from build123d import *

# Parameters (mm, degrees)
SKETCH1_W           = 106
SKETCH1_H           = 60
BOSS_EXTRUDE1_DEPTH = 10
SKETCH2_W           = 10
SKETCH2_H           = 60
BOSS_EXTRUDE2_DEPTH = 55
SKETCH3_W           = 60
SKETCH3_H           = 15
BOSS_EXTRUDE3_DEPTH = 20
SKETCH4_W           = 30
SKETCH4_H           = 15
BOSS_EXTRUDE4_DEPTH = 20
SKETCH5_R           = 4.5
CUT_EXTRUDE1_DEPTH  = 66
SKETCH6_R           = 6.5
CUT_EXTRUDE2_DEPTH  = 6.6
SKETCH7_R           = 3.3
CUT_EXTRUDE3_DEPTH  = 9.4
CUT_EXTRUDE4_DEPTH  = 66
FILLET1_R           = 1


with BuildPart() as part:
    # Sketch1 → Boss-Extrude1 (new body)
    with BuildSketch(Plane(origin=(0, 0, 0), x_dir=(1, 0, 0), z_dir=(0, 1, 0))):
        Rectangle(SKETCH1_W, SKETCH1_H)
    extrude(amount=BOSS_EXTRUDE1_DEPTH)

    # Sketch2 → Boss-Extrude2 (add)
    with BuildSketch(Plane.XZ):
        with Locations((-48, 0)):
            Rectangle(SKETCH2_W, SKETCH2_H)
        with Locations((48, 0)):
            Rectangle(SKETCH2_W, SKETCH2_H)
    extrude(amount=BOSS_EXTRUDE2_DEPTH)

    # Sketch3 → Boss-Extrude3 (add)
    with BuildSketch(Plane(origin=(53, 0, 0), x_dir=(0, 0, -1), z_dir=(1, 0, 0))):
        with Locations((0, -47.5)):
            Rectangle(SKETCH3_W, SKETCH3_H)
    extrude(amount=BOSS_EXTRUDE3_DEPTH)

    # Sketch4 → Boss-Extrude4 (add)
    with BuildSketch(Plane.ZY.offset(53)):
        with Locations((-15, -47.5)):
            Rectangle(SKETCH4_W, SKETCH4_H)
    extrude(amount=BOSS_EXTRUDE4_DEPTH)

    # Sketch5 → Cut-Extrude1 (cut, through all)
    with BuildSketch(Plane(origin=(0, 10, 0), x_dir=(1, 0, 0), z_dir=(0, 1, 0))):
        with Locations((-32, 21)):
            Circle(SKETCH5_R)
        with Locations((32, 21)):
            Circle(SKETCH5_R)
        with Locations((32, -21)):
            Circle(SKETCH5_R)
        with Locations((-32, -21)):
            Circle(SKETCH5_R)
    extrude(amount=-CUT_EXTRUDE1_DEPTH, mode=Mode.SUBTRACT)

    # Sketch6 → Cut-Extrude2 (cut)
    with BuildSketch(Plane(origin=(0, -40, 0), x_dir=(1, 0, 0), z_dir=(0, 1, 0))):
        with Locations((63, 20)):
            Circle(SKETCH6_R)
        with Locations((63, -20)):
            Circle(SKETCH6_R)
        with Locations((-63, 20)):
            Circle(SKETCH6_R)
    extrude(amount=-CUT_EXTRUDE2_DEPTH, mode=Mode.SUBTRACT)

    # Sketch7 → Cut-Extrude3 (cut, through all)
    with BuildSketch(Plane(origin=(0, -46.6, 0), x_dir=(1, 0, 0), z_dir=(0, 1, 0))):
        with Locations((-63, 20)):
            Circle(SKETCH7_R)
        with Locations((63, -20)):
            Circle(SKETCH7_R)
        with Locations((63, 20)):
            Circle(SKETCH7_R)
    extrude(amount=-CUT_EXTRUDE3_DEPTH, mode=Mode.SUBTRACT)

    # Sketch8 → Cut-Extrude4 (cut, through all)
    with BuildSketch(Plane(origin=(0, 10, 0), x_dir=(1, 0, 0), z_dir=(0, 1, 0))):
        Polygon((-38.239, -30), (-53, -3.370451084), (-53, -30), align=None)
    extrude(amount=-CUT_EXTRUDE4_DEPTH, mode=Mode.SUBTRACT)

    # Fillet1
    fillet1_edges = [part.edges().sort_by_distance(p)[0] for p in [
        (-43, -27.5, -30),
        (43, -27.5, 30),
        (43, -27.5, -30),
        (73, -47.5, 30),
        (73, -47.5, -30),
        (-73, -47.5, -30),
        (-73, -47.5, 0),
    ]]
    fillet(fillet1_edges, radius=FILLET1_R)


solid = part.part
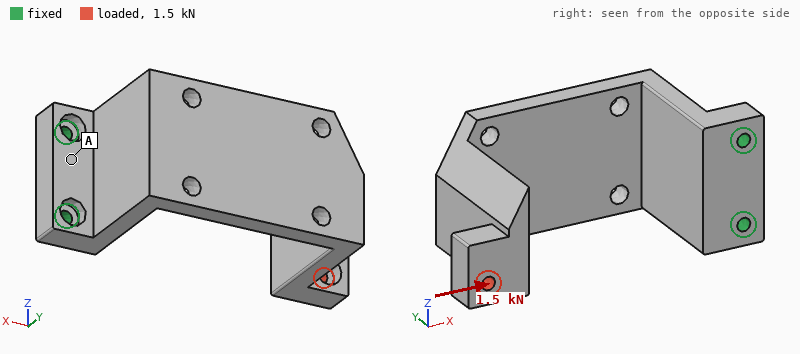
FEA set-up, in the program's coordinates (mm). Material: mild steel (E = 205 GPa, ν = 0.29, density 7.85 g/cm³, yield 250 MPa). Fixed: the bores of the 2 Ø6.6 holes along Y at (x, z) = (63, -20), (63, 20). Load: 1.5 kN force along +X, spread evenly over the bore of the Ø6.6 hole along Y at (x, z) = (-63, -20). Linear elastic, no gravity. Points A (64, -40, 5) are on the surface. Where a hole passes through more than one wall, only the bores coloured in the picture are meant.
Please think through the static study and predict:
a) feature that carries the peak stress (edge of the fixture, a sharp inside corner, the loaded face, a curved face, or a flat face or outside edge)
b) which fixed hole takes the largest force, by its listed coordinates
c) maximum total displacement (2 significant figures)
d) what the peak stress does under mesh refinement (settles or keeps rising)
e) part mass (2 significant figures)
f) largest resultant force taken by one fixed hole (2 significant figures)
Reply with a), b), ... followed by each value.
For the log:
a) a sharp inside corner
b) (63, -20)
c) 1.2 mm
d) keeps rising
e) 1.1 kg
f) 1.4 kN
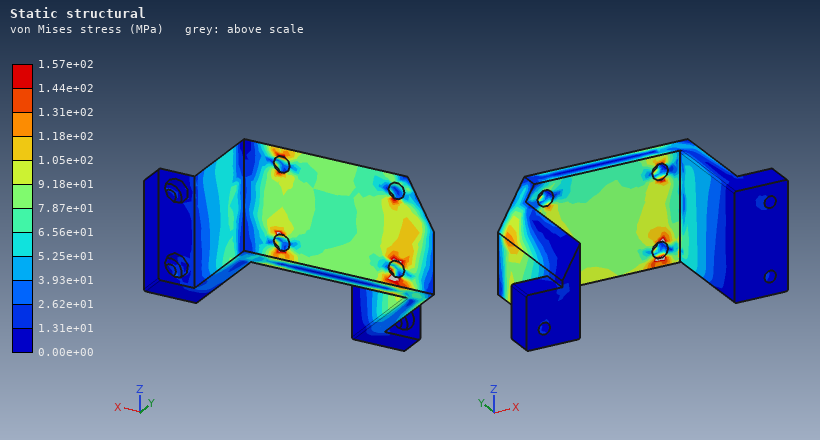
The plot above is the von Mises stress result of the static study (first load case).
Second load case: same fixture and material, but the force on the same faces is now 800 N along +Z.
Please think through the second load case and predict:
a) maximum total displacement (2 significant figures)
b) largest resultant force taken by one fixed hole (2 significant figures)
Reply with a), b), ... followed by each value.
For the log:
a) 0.52 mm
b) 2.3 kN
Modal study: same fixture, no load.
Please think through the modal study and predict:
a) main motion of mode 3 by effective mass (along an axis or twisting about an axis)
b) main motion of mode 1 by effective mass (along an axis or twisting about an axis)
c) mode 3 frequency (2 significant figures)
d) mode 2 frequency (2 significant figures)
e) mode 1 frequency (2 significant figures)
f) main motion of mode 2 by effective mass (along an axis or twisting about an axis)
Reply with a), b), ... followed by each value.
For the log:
a) along X
b) along Y
c) 710 Hz
d) 450 Hz
e) 260 Hz
f) along Z
